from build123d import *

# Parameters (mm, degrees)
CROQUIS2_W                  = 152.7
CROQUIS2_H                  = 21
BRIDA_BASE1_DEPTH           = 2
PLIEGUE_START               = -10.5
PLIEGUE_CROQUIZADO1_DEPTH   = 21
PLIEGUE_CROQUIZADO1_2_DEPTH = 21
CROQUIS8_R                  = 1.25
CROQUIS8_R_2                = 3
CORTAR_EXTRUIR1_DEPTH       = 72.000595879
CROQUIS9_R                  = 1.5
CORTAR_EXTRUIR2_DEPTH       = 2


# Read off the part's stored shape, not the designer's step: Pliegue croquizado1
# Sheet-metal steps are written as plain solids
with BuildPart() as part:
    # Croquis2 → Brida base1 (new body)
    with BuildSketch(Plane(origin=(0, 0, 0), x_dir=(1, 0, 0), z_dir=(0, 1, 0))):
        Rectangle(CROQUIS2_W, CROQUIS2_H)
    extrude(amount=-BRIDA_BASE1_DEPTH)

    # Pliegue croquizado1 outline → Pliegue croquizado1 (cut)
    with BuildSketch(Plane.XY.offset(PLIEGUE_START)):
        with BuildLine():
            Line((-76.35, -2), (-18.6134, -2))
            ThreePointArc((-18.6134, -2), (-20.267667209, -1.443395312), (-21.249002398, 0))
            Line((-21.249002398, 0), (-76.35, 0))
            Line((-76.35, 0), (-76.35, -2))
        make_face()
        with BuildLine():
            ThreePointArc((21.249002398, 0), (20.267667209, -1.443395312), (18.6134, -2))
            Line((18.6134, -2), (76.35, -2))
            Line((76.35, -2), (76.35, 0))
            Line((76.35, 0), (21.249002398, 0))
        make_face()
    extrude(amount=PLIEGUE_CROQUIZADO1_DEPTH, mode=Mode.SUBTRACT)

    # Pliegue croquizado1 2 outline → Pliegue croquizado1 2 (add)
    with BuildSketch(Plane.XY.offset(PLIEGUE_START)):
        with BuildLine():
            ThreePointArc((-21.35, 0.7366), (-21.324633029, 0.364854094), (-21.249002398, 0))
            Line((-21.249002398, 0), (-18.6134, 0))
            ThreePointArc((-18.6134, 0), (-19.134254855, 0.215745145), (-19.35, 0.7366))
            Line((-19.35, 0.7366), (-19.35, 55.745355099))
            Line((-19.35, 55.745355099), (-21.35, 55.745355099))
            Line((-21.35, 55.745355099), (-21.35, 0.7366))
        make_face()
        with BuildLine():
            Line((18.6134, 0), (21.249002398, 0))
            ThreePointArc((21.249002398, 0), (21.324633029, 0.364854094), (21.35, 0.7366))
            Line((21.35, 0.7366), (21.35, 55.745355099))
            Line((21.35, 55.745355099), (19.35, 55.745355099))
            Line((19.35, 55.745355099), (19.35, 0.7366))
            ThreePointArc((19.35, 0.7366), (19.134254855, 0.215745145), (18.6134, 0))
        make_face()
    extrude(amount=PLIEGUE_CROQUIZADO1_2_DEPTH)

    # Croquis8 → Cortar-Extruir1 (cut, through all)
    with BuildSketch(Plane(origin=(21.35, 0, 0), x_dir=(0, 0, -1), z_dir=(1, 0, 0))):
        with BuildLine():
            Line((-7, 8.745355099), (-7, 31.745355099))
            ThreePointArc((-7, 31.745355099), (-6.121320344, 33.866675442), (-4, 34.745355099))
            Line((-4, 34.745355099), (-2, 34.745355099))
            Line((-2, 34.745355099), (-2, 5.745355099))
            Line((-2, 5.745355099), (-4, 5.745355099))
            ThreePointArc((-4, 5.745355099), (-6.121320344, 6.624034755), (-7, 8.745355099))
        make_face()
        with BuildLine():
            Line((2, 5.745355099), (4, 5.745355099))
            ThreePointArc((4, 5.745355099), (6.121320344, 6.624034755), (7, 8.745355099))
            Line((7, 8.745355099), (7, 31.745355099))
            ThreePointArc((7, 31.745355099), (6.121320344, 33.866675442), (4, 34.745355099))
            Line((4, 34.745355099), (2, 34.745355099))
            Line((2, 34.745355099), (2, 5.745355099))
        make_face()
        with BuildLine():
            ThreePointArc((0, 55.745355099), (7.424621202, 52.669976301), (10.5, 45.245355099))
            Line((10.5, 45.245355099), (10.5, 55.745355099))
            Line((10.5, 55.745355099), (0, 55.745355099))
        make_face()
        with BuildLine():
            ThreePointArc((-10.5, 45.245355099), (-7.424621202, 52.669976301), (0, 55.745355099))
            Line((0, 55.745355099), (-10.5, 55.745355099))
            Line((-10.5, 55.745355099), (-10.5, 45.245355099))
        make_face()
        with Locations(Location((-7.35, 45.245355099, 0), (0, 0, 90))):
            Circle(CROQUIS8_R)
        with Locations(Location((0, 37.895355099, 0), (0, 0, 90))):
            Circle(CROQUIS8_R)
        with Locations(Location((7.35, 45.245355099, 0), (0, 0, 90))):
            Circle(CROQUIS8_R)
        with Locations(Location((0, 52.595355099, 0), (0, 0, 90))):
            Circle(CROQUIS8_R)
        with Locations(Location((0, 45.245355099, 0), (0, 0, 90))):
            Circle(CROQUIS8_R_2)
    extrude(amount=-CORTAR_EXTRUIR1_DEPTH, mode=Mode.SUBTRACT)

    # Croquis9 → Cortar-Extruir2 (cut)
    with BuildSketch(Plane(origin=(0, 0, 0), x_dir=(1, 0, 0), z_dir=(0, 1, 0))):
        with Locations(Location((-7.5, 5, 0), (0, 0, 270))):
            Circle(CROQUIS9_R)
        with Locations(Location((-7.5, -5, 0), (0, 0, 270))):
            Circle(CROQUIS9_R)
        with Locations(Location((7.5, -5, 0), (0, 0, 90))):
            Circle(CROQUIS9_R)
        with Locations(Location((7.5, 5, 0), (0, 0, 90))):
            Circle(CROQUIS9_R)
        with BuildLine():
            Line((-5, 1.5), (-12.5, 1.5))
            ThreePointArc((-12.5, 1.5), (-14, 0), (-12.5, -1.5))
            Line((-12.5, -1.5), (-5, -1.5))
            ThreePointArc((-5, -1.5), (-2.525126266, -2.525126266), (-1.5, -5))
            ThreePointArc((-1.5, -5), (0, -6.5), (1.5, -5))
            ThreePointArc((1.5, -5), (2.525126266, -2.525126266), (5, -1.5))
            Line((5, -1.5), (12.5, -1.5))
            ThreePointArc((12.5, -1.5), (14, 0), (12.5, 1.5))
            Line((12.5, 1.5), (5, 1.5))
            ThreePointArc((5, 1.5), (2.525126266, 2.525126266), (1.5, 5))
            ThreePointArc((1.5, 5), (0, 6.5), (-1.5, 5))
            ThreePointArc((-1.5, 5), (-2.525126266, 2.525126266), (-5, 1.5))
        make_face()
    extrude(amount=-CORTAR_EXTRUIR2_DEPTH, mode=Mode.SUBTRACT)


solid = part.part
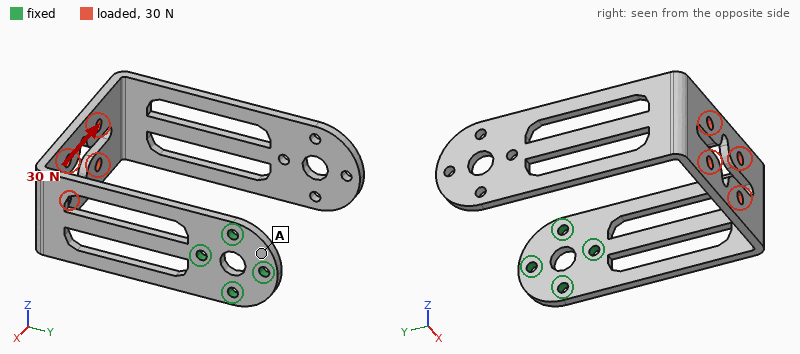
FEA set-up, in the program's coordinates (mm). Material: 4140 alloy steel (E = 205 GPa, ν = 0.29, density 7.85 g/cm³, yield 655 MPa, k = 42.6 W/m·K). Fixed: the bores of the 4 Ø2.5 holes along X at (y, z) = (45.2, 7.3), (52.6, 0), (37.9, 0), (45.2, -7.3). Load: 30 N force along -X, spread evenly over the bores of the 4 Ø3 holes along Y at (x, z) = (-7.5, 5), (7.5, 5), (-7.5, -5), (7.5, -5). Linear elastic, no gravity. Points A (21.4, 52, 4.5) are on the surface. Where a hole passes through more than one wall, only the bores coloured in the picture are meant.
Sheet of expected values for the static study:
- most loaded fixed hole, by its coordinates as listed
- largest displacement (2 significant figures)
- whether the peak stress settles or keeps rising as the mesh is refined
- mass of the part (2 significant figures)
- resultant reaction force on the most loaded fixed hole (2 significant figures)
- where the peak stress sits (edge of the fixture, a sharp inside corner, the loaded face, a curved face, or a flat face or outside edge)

(37.9, 0)
0.74 mm
keeps rising
36 g
95 N
edge of the fixture
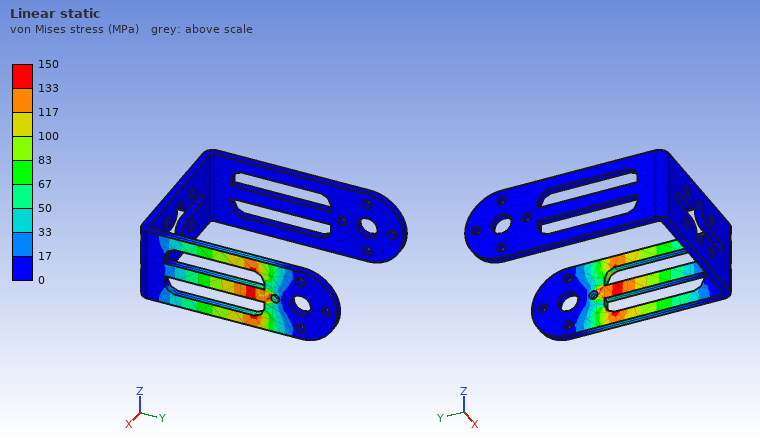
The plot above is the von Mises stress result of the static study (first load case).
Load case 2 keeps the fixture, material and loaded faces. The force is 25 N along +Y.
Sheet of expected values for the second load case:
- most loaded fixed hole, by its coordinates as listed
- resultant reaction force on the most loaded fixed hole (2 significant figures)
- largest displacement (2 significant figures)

(37.9, 0)
35 N
0.80 mm
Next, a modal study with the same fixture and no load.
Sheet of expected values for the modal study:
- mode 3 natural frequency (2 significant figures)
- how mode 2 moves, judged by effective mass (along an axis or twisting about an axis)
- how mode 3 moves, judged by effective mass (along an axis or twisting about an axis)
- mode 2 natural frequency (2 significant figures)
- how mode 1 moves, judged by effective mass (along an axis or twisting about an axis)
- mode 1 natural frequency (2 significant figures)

310 Hz
along Z
along X
200 Hz
along Y
150 Hz
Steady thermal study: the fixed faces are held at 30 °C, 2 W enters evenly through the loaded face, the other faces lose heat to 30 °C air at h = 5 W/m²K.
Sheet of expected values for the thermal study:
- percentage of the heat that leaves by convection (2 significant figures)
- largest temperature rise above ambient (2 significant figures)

51 %
54 K
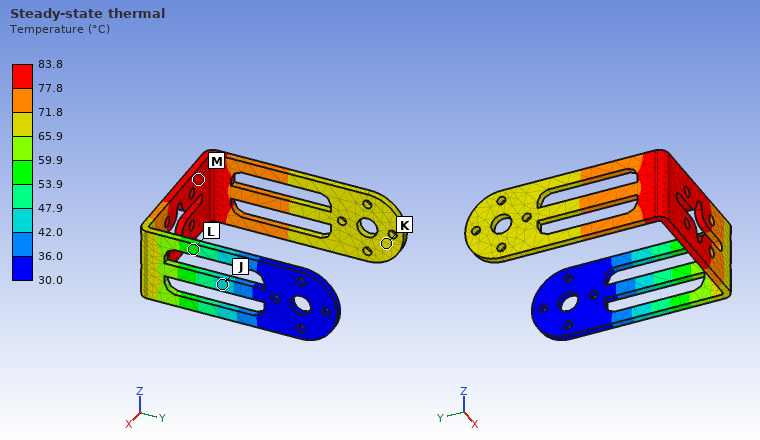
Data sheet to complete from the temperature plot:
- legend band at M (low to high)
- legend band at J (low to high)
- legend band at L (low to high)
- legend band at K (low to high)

77.8 to 83.8 °C
42.0 to 47.9 °C
53.9 to 59.9 °C
65.9 to 71.8 °C
